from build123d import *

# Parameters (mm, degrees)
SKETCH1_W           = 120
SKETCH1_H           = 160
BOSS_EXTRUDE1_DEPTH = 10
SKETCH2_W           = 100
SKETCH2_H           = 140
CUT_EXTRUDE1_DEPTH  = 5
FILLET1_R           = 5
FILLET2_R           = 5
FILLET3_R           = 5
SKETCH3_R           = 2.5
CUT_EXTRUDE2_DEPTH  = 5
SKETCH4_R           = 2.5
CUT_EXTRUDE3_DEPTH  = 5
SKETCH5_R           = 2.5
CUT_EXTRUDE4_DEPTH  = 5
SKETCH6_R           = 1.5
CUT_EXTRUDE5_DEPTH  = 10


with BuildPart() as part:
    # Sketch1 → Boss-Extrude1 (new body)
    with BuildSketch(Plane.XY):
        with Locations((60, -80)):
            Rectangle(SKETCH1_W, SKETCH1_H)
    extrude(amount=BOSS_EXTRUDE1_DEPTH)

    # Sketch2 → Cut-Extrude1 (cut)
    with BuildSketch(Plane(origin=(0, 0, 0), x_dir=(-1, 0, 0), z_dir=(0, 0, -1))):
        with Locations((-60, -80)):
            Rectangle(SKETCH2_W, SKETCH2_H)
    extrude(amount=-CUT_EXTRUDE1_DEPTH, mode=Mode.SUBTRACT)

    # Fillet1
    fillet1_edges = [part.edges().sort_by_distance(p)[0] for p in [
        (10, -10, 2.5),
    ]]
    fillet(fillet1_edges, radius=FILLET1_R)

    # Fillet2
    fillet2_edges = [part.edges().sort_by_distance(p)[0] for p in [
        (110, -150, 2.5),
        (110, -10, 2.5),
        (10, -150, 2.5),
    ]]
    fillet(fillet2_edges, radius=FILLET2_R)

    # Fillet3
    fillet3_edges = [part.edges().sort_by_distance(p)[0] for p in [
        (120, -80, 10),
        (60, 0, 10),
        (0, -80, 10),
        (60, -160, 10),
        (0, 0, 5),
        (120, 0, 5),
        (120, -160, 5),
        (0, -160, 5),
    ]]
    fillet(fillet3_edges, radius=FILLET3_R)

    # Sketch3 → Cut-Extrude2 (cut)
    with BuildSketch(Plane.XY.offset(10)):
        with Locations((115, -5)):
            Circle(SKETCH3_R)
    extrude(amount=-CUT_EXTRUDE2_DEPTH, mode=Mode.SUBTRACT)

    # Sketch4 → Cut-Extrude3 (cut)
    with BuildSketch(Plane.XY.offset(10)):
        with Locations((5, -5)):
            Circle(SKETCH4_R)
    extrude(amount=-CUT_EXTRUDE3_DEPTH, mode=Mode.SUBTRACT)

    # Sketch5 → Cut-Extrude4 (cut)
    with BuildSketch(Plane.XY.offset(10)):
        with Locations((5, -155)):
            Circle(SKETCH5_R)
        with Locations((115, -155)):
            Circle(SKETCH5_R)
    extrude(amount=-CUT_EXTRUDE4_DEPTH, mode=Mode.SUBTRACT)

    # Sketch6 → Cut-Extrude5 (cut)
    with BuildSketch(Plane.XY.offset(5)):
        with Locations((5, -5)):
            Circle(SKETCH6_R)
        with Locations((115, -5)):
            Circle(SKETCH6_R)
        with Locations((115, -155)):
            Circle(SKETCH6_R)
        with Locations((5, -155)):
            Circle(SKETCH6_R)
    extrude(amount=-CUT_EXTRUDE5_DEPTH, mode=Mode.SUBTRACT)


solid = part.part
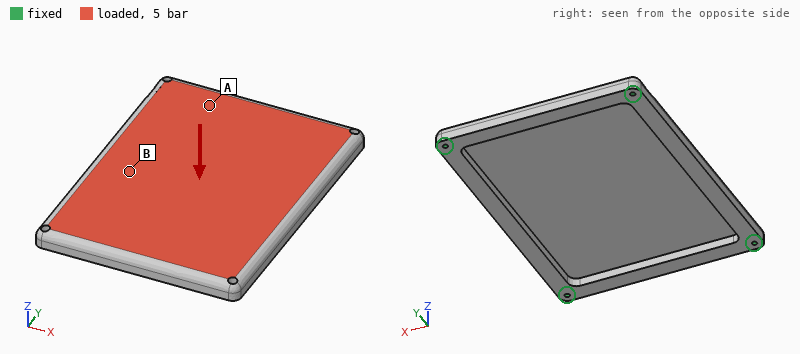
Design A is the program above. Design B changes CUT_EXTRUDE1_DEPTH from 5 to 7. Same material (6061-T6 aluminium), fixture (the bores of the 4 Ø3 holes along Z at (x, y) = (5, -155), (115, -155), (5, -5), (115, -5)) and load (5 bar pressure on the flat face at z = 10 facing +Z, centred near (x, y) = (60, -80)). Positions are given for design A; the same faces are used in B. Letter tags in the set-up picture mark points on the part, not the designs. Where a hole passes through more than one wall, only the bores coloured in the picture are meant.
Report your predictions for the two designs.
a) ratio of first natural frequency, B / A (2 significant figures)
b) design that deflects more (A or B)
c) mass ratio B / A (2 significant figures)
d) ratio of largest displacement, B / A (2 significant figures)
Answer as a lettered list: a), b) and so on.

a) 0.98
b) B
c) 0.76
d) 1.9
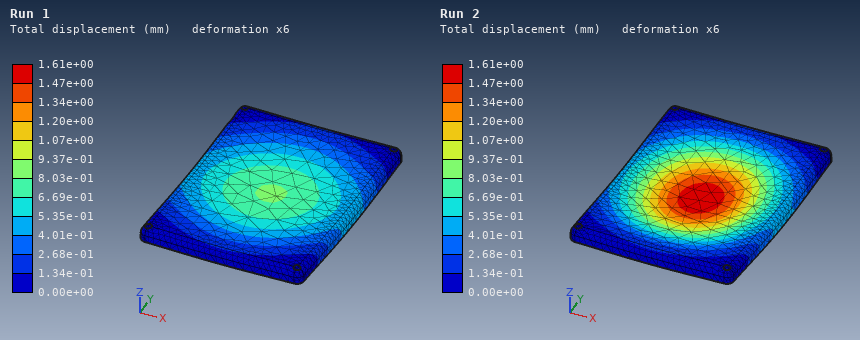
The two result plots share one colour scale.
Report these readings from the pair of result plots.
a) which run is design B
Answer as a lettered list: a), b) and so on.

a) Run 2
